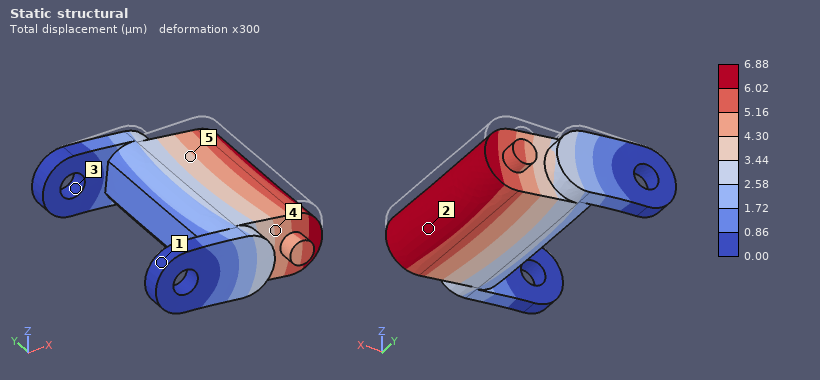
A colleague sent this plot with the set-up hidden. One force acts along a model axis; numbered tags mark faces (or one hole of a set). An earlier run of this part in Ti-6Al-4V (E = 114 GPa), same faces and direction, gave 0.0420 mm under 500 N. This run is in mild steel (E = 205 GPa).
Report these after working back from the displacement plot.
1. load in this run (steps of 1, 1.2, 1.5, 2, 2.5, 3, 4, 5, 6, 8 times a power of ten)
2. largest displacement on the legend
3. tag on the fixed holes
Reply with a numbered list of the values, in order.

1. 150 N
2. 6.88 µm
3. 3
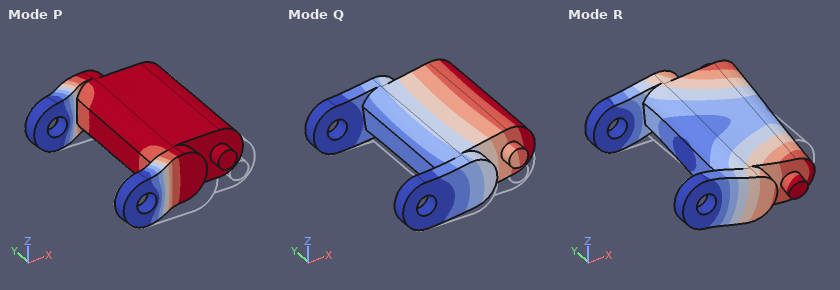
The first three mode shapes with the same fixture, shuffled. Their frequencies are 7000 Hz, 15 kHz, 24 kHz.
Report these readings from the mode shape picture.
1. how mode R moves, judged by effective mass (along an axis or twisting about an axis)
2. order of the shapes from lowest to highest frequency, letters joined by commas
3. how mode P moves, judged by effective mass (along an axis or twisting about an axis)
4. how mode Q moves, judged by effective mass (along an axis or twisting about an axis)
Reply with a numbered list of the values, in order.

1. twisting about X
2. Q, P, R
3. along Y
4. along Z
